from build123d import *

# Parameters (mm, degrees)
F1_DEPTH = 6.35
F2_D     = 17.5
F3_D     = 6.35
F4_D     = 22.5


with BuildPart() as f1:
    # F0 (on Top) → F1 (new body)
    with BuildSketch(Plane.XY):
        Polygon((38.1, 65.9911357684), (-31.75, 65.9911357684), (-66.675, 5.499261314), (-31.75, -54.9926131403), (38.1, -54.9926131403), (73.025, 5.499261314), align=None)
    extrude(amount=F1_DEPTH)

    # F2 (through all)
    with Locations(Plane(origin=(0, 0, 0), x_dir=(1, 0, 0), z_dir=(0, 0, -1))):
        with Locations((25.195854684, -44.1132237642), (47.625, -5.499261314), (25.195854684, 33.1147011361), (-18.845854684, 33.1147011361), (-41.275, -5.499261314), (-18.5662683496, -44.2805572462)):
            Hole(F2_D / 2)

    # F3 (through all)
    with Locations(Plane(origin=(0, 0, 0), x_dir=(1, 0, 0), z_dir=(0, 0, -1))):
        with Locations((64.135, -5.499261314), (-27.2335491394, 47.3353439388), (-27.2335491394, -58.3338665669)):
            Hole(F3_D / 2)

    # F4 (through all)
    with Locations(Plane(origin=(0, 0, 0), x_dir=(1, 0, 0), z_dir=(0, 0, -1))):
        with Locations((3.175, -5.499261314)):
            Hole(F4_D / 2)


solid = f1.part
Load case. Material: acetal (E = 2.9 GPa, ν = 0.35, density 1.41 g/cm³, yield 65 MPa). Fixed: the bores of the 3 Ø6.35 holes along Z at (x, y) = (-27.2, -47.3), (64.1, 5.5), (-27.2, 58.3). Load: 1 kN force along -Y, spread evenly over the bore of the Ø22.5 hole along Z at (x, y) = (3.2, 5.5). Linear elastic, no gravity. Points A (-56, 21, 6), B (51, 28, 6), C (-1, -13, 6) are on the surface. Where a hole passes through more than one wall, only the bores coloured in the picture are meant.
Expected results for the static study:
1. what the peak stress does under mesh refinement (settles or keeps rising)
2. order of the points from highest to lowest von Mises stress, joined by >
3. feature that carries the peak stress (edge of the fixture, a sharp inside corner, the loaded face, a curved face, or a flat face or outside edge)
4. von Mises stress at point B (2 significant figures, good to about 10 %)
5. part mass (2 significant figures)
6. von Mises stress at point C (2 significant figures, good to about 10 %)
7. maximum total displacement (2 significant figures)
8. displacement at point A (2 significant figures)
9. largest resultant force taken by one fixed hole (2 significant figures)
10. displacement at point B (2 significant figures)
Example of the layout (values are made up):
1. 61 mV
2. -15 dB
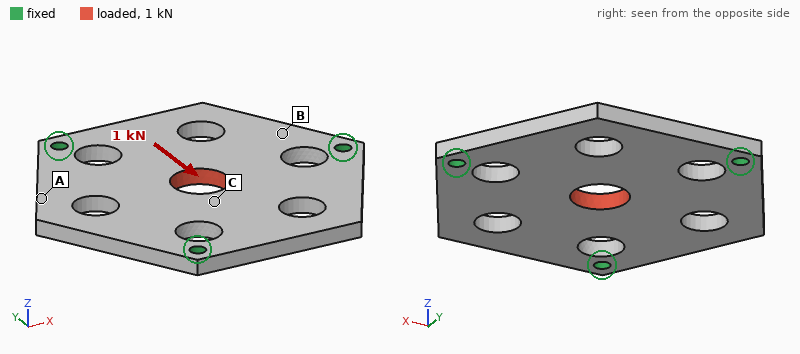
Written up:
1. keeps rising
2. C > B > A
3. edge of the fixture
4. 1.5 MPa
5. 96 g
6. 2.4 MPa
7. 79 µm
8. 19 µm
9. 350 N
10. 34 µm
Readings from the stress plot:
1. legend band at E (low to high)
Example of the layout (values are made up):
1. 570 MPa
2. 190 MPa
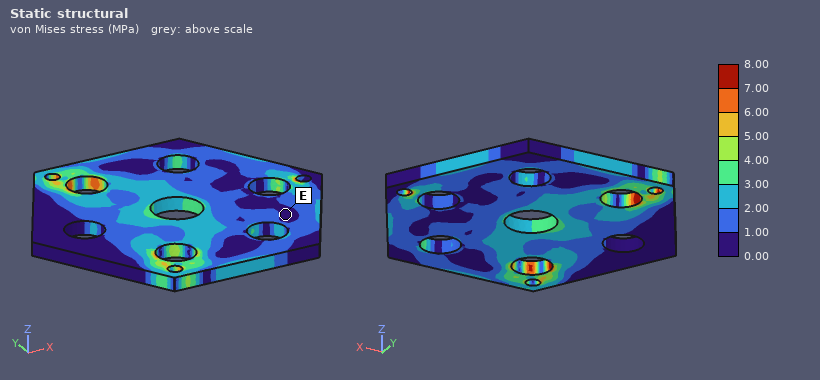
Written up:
1. 0.00 to 1.00 MPa
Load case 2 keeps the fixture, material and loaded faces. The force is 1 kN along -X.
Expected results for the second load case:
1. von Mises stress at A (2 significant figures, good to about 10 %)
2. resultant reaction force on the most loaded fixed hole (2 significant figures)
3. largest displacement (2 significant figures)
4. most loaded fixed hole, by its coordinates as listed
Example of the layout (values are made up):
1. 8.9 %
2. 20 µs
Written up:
1. 1.8 MPa
2. 360 N
3. 81 µm
4. (64.1, 5.5)
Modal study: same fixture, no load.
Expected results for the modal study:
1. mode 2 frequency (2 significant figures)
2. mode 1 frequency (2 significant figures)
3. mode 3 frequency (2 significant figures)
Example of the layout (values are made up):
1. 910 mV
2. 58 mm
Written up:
1. 590 Hz
2. 580 Hz
3. 590 Hz
